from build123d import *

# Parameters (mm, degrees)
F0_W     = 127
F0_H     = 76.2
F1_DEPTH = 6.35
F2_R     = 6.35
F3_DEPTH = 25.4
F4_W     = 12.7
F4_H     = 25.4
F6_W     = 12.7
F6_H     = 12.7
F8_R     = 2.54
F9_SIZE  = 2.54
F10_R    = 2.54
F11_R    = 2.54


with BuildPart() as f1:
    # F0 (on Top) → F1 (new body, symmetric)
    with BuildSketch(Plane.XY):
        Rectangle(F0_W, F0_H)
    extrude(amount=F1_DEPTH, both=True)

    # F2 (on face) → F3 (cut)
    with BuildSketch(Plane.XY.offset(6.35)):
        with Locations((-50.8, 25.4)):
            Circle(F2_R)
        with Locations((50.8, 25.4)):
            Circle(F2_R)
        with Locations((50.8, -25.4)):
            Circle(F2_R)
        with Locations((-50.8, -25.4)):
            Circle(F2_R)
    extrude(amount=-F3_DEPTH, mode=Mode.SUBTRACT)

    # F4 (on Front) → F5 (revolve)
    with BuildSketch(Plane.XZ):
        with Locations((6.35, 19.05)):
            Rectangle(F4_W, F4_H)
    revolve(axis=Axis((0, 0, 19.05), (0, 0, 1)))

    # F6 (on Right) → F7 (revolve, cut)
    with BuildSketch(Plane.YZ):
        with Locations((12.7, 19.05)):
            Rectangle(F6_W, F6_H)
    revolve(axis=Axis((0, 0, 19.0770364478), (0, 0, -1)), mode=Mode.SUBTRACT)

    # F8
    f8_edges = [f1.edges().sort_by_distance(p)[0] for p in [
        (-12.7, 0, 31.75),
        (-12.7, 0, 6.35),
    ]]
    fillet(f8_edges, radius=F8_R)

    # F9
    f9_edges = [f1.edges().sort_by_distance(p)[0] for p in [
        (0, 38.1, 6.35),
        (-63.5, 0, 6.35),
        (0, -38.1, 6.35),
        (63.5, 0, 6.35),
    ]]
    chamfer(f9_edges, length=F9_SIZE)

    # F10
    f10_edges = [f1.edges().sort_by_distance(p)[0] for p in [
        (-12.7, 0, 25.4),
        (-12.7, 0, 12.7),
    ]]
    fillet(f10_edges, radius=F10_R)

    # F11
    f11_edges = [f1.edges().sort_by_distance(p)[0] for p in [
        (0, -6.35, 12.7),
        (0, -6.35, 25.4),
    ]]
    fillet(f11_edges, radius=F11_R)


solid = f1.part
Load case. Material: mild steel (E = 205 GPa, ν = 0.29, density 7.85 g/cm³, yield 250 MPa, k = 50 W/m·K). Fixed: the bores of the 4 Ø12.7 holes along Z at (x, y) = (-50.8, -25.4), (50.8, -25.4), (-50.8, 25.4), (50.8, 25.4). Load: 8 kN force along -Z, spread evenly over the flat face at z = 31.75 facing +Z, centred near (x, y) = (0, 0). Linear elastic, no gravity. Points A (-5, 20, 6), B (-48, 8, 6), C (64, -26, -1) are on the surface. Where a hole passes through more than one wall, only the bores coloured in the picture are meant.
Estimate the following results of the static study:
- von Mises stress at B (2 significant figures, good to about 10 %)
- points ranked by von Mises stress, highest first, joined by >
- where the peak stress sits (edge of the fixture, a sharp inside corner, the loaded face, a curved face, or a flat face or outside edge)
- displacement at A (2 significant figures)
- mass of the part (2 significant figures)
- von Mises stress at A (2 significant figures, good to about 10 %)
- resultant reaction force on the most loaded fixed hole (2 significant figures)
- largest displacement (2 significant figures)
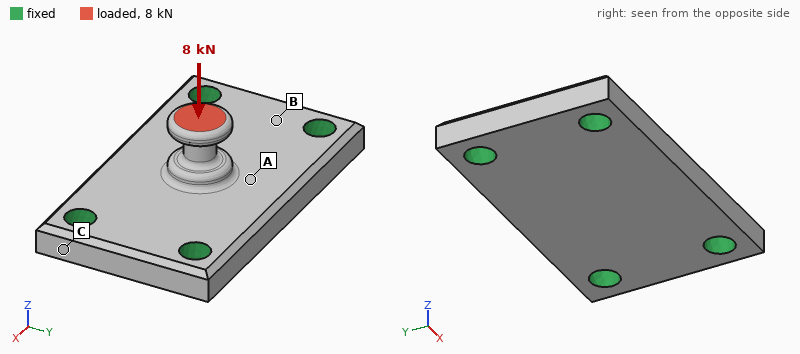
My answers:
15 MPa
A > B > C
a curved face
14 µm
970 g
25 MPa
2.0 kN
22 µm
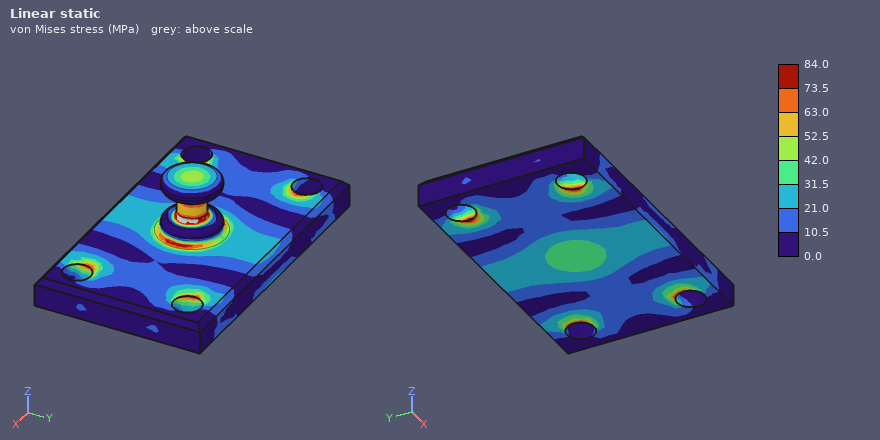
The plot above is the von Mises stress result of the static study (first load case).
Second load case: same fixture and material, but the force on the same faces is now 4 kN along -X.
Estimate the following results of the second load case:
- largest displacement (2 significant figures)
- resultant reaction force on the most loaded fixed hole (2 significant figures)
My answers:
72 µm
1.4 kN
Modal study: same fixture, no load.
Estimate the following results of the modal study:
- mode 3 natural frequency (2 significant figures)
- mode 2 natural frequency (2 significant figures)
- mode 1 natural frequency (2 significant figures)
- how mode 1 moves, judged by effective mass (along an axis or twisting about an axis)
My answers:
8700 Hz
7100 Hz
6000 Hz
along Z
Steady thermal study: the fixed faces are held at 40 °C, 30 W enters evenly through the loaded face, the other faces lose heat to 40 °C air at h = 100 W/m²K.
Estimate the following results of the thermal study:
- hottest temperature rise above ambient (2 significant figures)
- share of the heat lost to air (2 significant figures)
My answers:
78 K
52 %
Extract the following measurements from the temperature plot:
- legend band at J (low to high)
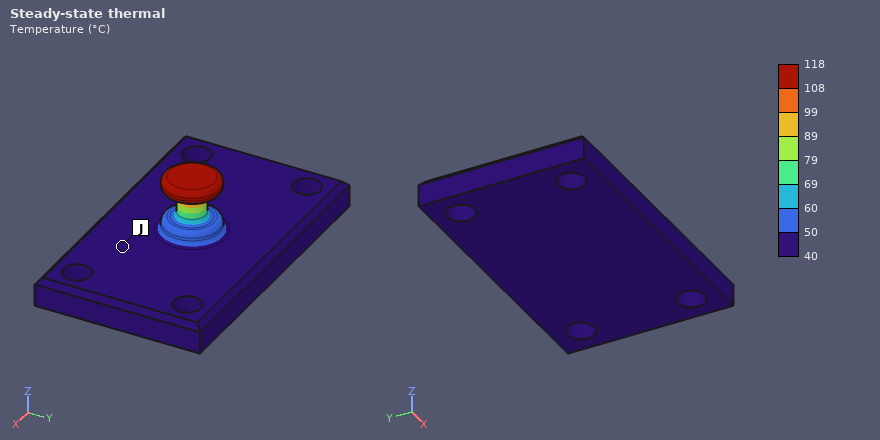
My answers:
40 to 50 °C
